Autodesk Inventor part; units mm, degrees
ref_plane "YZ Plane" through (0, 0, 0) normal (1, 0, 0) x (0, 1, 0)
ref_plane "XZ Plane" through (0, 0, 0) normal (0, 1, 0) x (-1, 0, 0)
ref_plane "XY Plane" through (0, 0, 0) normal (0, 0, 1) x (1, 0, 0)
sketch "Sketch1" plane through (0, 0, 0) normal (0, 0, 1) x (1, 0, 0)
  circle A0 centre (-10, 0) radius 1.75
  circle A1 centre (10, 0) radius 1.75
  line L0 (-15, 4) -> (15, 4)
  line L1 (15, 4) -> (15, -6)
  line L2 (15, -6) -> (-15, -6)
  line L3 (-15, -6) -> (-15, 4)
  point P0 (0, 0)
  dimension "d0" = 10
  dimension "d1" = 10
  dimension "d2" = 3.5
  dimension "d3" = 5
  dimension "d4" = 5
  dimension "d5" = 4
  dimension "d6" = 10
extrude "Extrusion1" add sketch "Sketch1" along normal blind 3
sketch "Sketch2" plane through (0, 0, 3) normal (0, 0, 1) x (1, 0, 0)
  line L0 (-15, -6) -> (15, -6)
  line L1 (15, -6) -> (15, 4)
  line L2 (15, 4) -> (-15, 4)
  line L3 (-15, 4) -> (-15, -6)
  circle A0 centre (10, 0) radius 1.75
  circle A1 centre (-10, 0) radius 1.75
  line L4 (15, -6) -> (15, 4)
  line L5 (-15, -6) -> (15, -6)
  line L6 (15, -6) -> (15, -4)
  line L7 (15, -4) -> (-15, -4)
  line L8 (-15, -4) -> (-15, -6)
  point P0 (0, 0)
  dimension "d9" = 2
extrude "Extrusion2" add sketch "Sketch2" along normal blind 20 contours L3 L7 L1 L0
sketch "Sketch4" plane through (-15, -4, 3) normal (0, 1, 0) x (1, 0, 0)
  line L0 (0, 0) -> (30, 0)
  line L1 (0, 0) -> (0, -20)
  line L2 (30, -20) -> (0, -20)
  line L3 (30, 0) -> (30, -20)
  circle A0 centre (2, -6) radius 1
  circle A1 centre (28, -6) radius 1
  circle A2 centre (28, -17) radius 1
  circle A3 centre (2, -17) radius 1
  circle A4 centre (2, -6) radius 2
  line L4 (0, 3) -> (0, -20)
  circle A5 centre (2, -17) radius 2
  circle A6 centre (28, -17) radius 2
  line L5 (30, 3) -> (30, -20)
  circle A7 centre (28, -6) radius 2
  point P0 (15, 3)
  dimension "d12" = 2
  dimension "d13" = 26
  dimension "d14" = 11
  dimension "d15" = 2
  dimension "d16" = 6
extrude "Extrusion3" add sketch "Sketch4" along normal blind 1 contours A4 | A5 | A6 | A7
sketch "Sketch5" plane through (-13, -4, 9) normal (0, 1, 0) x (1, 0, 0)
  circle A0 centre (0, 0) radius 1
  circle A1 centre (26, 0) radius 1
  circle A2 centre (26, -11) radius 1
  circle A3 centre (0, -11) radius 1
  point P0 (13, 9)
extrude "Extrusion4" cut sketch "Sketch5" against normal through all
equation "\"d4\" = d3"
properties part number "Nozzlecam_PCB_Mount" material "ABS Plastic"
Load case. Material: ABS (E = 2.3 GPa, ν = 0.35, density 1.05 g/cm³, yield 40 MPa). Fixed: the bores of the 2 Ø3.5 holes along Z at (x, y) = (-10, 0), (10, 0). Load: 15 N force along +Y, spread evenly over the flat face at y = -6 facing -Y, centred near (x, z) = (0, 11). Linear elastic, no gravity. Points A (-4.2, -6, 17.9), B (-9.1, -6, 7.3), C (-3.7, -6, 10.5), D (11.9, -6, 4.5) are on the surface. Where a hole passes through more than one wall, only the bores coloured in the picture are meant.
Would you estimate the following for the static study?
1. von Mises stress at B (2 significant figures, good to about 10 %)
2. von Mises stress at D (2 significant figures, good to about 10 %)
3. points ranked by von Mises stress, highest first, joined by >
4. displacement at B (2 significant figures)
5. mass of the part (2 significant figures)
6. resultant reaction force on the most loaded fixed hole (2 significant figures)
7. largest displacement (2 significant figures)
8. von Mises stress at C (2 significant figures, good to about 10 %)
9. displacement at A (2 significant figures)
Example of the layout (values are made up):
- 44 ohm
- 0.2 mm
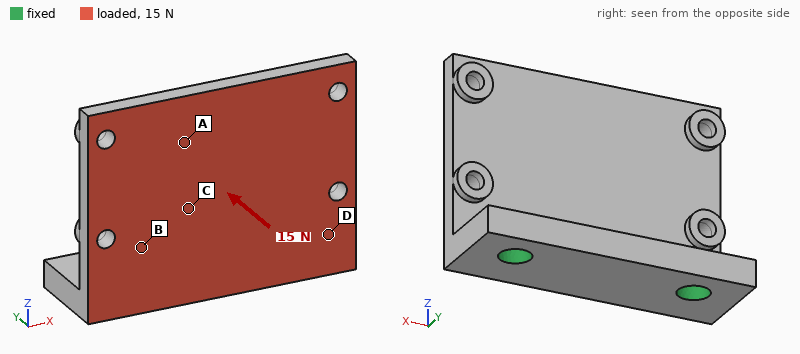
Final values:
- 3.7 MPa
- 4.9 MPa
- D > B > C > A
- 0.063 mm
- 2.2 g
- 7.6 N
- 0.40 mm
- 2.2 MPa
- 0.28 mm
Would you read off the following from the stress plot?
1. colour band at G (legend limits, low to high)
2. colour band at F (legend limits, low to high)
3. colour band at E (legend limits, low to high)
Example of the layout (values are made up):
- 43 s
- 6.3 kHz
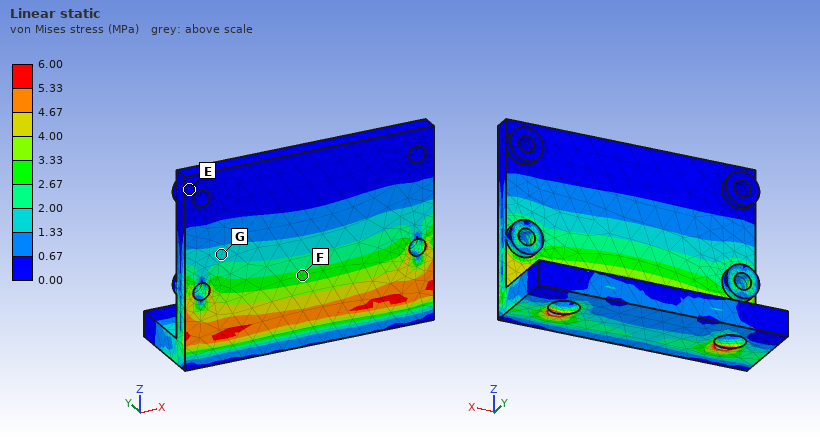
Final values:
- 1.33 to 2.00 MPa
- 2.67 to 3.33 MPa
- 0.00 to 0.67 MPa
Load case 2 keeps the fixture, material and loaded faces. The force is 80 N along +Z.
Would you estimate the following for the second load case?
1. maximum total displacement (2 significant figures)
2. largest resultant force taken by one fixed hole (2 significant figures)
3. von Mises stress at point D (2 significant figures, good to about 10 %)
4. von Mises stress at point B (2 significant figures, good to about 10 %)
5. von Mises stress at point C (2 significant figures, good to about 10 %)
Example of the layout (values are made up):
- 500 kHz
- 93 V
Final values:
- 0.41 mm
- 40 N
- 4.3 MPa
- 3.9 MPa
- 2.5 MPa
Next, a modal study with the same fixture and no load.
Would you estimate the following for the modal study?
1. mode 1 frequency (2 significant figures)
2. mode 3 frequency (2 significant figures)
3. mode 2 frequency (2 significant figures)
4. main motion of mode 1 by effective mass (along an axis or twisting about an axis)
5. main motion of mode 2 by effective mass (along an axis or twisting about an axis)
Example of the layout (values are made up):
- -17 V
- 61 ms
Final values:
- 1000 Hz
- 4600 Hz
- 1900 Hz
- along Y
- twisting about Z
